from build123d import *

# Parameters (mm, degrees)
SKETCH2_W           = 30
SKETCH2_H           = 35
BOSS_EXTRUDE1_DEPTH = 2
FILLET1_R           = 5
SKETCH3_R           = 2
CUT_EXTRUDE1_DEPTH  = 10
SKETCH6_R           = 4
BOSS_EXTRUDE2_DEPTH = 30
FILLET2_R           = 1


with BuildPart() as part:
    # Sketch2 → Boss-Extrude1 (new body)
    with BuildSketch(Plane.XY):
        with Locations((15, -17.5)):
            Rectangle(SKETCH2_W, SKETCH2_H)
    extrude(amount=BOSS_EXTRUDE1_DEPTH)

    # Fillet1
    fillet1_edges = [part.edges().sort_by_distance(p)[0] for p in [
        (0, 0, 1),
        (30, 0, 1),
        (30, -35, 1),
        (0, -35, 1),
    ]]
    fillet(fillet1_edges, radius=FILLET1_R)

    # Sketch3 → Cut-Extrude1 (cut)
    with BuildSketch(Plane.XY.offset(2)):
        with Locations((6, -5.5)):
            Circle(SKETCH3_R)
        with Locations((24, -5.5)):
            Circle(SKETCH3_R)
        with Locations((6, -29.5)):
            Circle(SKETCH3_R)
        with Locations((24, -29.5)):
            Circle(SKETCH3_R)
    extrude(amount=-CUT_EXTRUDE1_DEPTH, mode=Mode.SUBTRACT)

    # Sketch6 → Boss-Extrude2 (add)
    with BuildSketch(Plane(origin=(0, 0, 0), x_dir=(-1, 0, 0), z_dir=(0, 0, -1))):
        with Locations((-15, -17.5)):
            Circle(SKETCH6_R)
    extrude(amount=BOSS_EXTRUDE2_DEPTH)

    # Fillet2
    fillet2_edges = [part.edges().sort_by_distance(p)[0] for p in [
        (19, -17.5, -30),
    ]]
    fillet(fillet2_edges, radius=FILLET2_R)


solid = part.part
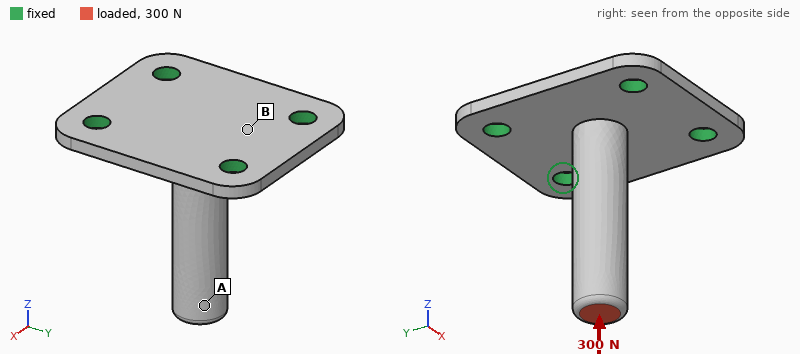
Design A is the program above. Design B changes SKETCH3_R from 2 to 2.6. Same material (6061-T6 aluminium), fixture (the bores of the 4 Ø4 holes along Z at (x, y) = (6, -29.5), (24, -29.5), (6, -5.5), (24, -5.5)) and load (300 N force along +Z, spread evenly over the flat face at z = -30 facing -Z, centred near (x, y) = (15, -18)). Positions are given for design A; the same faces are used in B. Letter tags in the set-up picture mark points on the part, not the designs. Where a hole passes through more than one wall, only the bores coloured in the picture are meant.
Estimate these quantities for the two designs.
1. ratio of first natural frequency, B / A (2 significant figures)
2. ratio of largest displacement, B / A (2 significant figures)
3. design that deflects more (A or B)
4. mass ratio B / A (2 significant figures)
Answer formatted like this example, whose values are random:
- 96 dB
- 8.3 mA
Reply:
- 1.0
- 0.87
- A
- 0.98
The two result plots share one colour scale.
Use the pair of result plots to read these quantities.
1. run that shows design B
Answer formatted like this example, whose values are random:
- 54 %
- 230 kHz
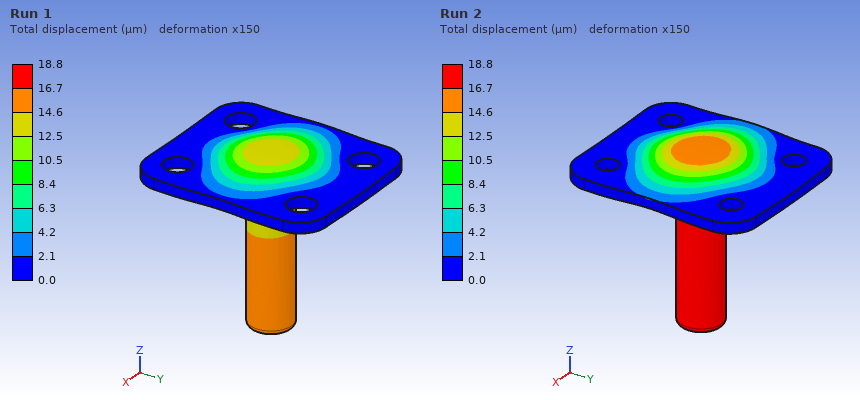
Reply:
- Run 1
